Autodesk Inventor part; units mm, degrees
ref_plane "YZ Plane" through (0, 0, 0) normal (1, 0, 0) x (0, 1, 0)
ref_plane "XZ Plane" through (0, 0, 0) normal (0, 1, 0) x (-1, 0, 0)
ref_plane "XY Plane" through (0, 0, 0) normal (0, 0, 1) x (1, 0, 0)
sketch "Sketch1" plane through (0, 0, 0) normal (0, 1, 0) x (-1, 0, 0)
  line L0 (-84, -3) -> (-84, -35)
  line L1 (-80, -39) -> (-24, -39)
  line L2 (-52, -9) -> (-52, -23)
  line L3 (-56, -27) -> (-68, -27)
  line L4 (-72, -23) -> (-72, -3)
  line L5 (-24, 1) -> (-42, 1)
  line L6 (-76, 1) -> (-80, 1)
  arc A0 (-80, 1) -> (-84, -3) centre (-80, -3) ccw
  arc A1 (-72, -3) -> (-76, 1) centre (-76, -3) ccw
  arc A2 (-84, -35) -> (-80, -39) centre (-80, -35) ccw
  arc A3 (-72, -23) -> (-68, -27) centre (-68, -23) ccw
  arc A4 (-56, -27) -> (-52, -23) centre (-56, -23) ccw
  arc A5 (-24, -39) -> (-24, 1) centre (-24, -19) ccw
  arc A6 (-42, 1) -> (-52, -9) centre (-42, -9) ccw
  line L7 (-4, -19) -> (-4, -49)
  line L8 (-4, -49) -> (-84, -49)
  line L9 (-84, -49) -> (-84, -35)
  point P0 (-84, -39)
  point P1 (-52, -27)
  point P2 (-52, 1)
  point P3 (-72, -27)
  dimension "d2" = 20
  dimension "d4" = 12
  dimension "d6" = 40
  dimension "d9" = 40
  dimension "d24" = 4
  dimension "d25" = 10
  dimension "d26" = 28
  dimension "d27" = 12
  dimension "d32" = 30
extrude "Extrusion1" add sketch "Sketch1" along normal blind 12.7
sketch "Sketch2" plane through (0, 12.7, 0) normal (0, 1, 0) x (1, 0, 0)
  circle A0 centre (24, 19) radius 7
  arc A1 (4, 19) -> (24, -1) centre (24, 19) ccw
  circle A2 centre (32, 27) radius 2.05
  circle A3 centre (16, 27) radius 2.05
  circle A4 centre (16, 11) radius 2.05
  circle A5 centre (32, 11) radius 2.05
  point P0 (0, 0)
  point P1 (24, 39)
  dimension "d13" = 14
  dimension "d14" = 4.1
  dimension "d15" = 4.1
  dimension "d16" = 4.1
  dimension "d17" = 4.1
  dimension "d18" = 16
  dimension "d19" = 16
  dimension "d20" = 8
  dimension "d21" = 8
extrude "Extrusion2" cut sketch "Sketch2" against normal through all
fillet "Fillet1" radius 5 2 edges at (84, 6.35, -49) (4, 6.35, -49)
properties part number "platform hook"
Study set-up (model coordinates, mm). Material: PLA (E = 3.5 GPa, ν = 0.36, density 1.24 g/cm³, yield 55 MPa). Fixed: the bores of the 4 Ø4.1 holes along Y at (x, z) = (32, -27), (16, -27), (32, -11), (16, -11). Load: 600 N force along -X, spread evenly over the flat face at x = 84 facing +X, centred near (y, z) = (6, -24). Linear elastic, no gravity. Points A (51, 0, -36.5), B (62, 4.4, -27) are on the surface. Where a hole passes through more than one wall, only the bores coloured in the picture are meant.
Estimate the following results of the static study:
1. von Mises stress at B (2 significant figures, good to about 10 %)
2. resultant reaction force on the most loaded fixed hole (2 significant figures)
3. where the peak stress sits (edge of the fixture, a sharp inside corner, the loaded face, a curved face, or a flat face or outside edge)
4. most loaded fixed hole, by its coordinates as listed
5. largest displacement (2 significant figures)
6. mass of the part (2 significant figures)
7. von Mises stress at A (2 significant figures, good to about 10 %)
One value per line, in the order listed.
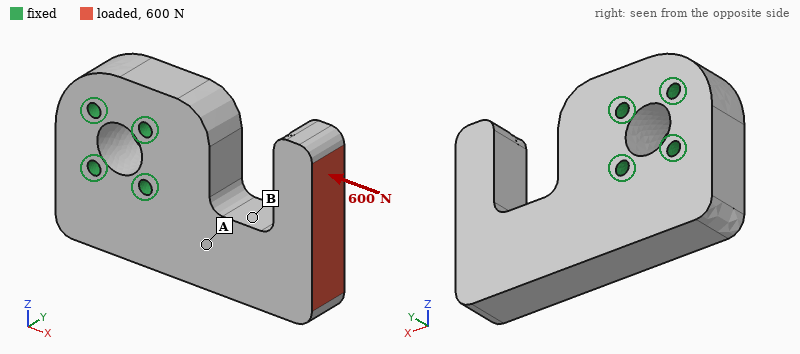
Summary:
11 MPa
440 N
a curved face
(32, -27)
0.53 mm
49 g
2.8 MPa
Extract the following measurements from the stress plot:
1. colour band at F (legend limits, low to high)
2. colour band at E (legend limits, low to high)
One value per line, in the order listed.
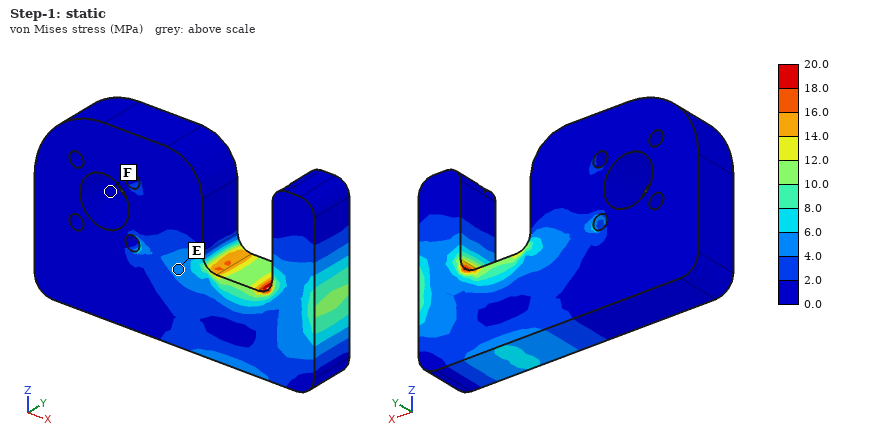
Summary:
0.0 to 2.0 MPa
4.0 to 6.0 MPa
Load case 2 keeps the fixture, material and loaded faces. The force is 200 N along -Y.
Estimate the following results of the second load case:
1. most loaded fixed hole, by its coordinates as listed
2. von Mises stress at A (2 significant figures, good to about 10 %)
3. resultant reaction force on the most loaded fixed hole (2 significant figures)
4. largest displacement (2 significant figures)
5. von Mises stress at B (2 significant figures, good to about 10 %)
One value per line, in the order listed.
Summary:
(32, -27)
11 MPa
280 N
0.94 mm
8.4 MPa
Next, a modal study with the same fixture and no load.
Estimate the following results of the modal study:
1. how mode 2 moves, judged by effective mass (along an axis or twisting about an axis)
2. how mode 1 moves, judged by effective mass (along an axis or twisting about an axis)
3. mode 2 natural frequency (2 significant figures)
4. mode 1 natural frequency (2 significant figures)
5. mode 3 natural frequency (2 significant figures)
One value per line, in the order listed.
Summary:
along Z
along Y
1600 Hz
910 Hz
1700 Hz
